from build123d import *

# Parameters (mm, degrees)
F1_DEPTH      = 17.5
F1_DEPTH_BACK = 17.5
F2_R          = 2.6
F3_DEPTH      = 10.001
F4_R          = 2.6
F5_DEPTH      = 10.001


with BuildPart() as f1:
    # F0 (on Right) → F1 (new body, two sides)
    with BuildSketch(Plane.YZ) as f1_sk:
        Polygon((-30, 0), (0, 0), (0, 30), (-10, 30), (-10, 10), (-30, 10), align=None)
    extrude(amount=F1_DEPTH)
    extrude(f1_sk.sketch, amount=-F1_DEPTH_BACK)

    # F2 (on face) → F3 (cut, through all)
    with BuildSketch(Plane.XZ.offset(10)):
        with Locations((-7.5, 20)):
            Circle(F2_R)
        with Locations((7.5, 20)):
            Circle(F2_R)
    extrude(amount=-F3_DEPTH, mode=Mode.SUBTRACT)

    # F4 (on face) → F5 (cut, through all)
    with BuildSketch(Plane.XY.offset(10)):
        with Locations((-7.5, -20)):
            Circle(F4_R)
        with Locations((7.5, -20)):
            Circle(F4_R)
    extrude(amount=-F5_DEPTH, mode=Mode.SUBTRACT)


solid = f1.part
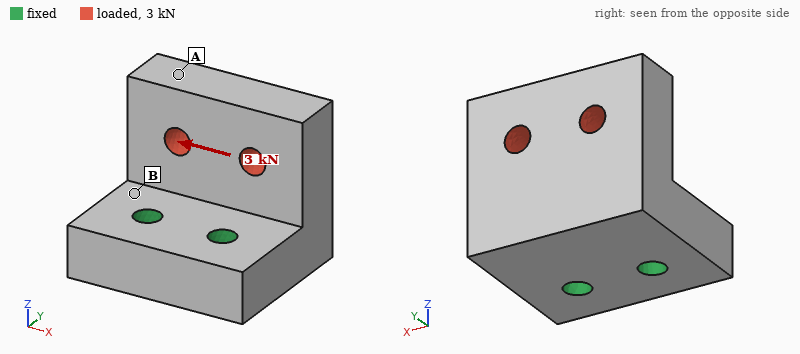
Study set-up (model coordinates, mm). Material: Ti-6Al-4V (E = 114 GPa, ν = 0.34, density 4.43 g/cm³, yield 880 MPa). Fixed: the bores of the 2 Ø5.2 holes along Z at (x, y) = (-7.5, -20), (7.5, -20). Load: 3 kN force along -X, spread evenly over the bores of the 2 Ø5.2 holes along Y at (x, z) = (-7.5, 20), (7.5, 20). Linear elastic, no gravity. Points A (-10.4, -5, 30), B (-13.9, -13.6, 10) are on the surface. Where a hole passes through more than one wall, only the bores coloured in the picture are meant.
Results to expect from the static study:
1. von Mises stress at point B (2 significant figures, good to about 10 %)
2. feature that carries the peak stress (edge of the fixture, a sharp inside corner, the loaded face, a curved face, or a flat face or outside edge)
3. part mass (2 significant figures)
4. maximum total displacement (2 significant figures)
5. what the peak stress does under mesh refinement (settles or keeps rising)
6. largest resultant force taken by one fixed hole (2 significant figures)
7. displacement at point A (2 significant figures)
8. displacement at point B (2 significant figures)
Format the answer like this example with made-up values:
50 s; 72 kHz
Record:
42 MPa; edge of the fixture; 74 g; 30 µm; keeps rising; 3.2 kN; 27 µm; 6.5 µm
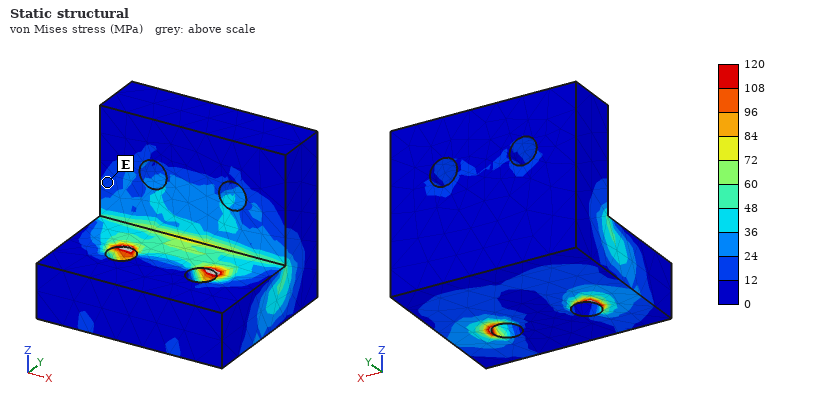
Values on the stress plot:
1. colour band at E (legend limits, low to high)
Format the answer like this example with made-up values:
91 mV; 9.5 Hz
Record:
12 to 24 MPa
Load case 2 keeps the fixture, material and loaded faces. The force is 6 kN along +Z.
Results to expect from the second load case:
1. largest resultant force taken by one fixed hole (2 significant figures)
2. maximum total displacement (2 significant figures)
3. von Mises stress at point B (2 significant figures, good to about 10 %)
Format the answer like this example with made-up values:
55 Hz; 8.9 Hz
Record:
3.0 kN; 65 µm; 68 MPa
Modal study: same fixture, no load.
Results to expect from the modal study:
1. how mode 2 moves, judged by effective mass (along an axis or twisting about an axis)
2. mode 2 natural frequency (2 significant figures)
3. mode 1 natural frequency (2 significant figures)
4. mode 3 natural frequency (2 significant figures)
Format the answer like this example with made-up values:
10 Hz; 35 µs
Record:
along X; 9900 Hz; 6800 Hz; 16 kHz
